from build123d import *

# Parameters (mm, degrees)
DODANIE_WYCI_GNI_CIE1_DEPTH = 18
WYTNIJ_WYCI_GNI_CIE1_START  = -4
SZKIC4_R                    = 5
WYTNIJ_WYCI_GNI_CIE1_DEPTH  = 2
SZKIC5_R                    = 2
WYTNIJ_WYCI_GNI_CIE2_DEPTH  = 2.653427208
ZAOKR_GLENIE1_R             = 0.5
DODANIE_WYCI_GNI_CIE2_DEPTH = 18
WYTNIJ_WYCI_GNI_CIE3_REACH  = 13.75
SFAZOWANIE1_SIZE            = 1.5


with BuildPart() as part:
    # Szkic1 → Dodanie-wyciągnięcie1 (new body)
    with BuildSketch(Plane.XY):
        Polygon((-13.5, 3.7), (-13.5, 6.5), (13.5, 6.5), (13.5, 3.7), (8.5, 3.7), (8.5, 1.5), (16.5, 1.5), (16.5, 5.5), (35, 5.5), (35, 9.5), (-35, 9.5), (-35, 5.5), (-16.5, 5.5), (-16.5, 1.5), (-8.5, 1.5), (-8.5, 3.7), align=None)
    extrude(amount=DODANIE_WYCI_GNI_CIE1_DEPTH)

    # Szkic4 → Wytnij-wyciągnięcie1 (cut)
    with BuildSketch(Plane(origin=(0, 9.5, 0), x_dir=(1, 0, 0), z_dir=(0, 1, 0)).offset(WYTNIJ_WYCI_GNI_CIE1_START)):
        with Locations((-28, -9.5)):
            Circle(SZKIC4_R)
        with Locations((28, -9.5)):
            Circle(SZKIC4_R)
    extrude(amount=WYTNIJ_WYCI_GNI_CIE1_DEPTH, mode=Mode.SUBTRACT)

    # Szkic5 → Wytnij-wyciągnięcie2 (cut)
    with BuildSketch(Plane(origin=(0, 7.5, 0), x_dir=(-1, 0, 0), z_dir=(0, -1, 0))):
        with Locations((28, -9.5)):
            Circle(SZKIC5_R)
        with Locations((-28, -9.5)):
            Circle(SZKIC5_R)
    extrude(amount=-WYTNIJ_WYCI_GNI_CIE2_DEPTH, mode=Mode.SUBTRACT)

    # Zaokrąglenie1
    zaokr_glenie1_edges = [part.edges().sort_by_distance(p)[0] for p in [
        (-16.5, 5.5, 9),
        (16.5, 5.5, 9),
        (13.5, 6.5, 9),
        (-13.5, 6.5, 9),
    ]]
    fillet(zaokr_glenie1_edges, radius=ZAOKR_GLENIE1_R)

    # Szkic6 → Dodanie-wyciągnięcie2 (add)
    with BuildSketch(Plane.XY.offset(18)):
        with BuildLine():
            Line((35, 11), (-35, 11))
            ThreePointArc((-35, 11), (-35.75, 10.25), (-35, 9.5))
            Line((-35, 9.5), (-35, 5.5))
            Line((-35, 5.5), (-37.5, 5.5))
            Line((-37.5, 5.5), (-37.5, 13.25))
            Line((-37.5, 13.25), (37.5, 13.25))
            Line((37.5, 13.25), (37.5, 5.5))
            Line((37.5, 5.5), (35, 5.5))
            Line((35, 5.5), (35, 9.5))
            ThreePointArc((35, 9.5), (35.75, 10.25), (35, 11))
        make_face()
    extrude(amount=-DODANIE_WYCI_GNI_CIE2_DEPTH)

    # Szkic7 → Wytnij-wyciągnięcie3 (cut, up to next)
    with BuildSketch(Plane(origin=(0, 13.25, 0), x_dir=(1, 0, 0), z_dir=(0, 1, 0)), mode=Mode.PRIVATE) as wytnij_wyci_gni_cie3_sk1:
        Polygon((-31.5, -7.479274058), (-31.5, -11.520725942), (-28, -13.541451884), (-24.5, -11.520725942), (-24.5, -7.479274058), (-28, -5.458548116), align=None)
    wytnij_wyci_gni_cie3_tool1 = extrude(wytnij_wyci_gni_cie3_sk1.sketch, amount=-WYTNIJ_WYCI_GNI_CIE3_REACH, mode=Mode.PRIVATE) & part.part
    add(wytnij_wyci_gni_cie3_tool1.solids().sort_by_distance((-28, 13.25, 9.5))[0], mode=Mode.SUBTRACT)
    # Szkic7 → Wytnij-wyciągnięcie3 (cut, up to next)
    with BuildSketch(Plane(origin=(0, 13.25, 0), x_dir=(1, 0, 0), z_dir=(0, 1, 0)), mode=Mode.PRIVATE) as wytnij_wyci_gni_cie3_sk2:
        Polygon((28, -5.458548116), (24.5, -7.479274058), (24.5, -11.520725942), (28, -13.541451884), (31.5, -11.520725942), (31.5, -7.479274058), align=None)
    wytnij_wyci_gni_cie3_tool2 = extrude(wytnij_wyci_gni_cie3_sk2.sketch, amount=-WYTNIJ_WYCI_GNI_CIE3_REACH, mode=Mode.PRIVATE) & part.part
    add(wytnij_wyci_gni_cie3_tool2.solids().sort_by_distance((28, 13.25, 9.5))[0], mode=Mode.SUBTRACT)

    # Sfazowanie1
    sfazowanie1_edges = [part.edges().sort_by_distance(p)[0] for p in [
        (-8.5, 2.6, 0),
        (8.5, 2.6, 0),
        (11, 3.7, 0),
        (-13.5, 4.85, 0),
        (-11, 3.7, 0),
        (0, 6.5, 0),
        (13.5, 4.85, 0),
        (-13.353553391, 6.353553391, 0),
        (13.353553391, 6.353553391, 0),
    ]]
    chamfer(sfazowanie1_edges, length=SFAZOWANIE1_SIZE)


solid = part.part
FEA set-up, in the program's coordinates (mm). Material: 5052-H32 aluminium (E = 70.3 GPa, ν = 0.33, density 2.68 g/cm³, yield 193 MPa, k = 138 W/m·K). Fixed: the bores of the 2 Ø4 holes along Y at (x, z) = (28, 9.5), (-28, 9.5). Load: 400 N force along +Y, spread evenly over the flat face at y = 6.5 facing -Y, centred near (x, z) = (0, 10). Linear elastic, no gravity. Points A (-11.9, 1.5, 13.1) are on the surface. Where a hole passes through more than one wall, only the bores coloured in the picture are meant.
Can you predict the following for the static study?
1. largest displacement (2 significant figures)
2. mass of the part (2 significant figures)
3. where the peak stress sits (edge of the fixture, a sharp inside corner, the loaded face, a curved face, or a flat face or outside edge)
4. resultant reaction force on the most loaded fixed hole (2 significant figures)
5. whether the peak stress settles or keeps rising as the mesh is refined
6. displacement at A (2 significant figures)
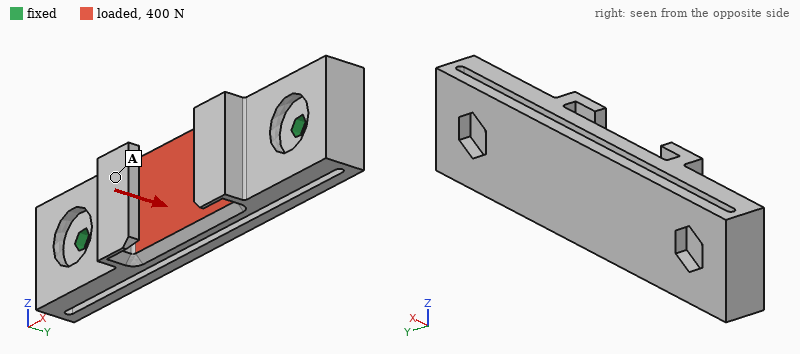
0.11 mm
22 g
edge of the fixture
200 N
keeps rising
0.081 mm
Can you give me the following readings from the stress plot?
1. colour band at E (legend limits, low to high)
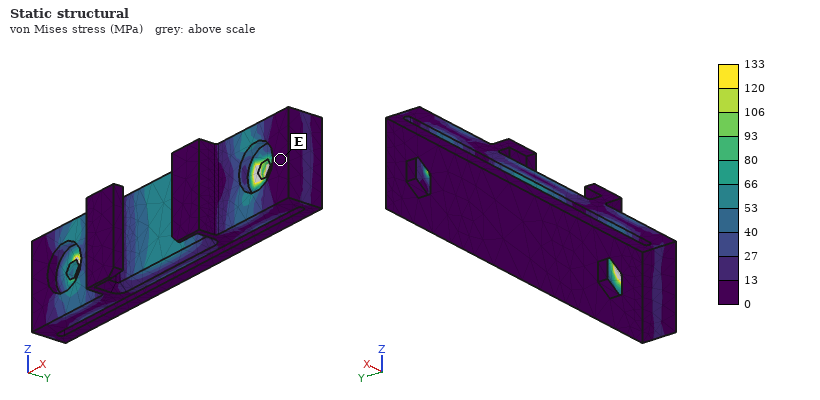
0 to 13 MPa
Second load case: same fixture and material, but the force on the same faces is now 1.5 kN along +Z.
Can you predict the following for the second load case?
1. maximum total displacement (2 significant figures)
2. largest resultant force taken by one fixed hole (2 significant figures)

61 µm
750 N
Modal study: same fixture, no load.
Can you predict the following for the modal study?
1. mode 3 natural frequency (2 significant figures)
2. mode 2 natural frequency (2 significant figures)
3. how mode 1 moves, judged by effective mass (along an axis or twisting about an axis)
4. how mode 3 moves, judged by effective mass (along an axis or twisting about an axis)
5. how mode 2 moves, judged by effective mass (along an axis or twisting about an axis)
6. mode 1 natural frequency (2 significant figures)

4800 Hz
4200 Hz
along Y
twisting about X
along Y
1900 Hz
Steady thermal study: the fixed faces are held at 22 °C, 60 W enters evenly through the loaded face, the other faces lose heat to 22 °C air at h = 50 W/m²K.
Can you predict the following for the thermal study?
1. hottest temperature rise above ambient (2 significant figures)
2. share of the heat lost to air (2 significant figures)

82 K
13 %
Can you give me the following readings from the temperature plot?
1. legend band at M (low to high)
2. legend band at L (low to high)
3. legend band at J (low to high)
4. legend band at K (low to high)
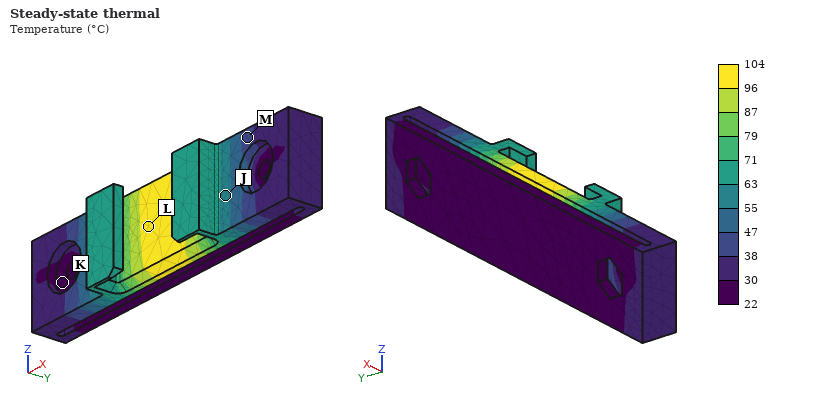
38 to 47 °C
96 to 104 °C
55 to 63 °C
22 to 30 °C
